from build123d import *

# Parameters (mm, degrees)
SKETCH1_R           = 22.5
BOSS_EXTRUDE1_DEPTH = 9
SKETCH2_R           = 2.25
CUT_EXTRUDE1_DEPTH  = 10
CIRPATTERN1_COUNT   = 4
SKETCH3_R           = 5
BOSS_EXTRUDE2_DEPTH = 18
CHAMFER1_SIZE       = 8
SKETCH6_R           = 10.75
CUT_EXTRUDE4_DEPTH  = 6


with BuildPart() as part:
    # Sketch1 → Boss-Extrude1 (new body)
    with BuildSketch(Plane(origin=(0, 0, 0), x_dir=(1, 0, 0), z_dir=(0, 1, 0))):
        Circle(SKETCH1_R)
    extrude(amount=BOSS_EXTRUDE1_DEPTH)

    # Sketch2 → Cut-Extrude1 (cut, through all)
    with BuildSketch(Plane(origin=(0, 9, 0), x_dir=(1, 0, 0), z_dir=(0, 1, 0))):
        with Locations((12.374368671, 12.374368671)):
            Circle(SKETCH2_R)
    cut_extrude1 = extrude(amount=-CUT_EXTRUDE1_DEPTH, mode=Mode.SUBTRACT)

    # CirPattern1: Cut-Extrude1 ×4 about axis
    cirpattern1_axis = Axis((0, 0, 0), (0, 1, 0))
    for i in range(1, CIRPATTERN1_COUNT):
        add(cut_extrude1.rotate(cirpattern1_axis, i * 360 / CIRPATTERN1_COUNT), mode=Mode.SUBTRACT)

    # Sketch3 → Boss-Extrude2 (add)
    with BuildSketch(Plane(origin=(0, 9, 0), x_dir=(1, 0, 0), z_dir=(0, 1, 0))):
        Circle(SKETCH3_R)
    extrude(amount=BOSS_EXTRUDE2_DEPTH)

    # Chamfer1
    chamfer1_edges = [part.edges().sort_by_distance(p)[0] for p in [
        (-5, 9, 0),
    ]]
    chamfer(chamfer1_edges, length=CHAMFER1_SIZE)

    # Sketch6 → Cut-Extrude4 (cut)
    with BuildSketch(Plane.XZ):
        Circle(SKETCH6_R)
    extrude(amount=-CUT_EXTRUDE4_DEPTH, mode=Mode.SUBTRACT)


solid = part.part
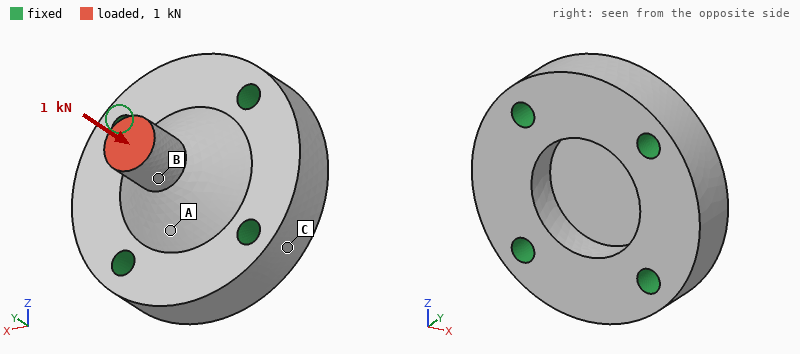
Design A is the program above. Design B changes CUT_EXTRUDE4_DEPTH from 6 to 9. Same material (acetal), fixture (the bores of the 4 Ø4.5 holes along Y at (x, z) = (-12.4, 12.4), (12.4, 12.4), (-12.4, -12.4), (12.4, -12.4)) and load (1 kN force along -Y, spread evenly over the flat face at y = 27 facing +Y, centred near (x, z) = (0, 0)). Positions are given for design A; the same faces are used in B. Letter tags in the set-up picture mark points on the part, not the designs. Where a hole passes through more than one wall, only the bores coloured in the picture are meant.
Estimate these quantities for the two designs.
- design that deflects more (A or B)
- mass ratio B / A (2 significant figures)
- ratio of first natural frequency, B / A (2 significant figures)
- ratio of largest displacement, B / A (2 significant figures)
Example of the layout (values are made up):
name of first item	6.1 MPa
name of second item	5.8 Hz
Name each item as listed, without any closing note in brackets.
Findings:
design that deflects more	B
mass ratio B / A	0.92
ratio of first natural frequency, B / A	0.95
ratio of largest displacement, B / A	1.2
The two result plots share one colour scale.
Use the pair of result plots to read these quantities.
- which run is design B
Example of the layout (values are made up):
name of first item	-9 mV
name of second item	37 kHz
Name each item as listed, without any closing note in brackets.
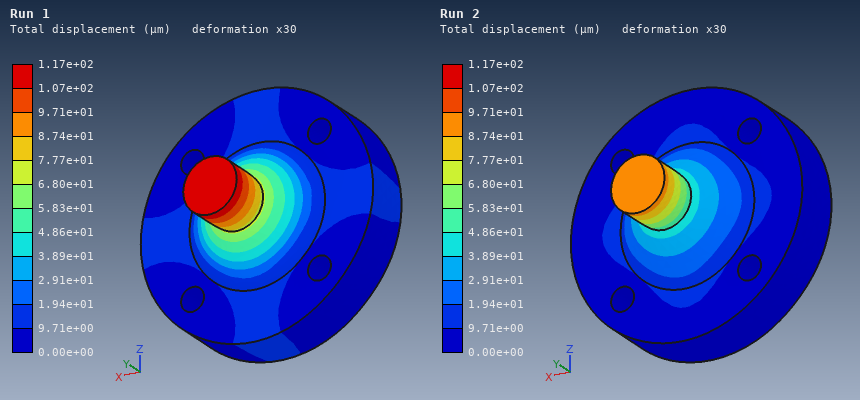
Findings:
which run is design B	Run 1
